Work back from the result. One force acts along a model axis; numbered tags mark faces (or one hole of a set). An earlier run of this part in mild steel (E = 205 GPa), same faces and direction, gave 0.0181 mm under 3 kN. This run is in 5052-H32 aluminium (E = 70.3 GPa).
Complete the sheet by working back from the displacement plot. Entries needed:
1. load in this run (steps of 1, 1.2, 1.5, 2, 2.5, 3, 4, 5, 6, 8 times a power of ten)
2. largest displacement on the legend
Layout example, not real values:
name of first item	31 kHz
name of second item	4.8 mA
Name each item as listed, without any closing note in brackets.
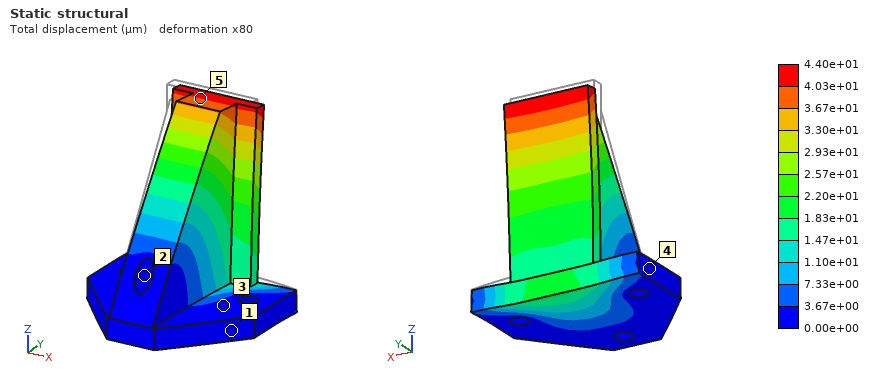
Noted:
load in this run	2.5 kN
largest displacement on the legend	4.40e+01 µm
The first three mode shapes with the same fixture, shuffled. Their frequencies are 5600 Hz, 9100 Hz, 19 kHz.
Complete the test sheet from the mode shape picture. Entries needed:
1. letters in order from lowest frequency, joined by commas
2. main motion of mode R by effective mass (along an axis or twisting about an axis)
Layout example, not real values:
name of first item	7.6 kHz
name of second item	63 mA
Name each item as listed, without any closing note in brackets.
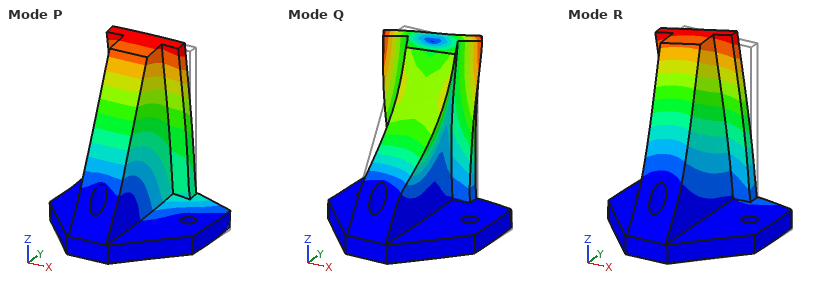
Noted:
letters in order from lowest frequency, joined by commas	R, P, Q
main motion of mode R by effective mass	along X
